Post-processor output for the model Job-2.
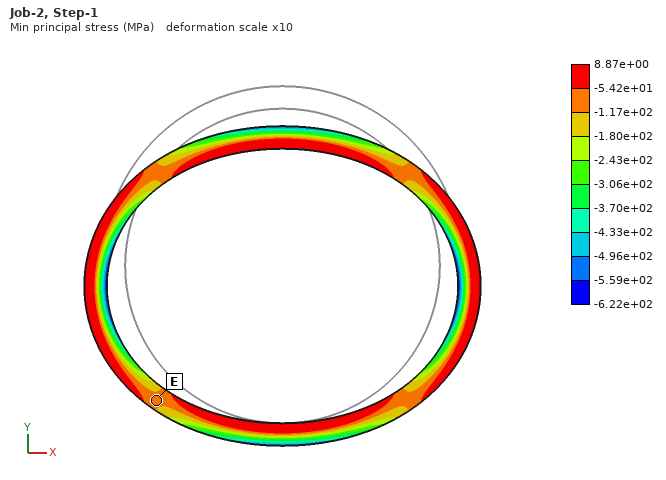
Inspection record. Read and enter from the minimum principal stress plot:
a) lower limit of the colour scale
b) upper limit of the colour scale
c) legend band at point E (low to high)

-6.22e+02 MPa
8.87e+00 MPa
-1.17e+02 to -5.42e+01 MPa
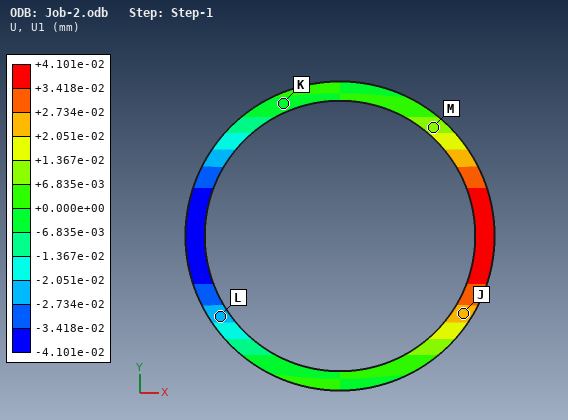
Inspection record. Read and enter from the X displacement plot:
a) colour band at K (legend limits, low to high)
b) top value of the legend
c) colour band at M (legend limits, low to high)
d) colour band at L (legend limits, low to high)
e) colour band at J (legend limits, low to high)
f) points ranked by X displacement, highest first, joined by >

-6.835e-03 to +0.000e+00 mm
+4.101e-02 mm
+6.835e-03 to +1.367e-02 mm
-2.734e-02 to -2.051e-02 mm
+2.051e-02 to +2.734e-02 mm
J > M > K > L
